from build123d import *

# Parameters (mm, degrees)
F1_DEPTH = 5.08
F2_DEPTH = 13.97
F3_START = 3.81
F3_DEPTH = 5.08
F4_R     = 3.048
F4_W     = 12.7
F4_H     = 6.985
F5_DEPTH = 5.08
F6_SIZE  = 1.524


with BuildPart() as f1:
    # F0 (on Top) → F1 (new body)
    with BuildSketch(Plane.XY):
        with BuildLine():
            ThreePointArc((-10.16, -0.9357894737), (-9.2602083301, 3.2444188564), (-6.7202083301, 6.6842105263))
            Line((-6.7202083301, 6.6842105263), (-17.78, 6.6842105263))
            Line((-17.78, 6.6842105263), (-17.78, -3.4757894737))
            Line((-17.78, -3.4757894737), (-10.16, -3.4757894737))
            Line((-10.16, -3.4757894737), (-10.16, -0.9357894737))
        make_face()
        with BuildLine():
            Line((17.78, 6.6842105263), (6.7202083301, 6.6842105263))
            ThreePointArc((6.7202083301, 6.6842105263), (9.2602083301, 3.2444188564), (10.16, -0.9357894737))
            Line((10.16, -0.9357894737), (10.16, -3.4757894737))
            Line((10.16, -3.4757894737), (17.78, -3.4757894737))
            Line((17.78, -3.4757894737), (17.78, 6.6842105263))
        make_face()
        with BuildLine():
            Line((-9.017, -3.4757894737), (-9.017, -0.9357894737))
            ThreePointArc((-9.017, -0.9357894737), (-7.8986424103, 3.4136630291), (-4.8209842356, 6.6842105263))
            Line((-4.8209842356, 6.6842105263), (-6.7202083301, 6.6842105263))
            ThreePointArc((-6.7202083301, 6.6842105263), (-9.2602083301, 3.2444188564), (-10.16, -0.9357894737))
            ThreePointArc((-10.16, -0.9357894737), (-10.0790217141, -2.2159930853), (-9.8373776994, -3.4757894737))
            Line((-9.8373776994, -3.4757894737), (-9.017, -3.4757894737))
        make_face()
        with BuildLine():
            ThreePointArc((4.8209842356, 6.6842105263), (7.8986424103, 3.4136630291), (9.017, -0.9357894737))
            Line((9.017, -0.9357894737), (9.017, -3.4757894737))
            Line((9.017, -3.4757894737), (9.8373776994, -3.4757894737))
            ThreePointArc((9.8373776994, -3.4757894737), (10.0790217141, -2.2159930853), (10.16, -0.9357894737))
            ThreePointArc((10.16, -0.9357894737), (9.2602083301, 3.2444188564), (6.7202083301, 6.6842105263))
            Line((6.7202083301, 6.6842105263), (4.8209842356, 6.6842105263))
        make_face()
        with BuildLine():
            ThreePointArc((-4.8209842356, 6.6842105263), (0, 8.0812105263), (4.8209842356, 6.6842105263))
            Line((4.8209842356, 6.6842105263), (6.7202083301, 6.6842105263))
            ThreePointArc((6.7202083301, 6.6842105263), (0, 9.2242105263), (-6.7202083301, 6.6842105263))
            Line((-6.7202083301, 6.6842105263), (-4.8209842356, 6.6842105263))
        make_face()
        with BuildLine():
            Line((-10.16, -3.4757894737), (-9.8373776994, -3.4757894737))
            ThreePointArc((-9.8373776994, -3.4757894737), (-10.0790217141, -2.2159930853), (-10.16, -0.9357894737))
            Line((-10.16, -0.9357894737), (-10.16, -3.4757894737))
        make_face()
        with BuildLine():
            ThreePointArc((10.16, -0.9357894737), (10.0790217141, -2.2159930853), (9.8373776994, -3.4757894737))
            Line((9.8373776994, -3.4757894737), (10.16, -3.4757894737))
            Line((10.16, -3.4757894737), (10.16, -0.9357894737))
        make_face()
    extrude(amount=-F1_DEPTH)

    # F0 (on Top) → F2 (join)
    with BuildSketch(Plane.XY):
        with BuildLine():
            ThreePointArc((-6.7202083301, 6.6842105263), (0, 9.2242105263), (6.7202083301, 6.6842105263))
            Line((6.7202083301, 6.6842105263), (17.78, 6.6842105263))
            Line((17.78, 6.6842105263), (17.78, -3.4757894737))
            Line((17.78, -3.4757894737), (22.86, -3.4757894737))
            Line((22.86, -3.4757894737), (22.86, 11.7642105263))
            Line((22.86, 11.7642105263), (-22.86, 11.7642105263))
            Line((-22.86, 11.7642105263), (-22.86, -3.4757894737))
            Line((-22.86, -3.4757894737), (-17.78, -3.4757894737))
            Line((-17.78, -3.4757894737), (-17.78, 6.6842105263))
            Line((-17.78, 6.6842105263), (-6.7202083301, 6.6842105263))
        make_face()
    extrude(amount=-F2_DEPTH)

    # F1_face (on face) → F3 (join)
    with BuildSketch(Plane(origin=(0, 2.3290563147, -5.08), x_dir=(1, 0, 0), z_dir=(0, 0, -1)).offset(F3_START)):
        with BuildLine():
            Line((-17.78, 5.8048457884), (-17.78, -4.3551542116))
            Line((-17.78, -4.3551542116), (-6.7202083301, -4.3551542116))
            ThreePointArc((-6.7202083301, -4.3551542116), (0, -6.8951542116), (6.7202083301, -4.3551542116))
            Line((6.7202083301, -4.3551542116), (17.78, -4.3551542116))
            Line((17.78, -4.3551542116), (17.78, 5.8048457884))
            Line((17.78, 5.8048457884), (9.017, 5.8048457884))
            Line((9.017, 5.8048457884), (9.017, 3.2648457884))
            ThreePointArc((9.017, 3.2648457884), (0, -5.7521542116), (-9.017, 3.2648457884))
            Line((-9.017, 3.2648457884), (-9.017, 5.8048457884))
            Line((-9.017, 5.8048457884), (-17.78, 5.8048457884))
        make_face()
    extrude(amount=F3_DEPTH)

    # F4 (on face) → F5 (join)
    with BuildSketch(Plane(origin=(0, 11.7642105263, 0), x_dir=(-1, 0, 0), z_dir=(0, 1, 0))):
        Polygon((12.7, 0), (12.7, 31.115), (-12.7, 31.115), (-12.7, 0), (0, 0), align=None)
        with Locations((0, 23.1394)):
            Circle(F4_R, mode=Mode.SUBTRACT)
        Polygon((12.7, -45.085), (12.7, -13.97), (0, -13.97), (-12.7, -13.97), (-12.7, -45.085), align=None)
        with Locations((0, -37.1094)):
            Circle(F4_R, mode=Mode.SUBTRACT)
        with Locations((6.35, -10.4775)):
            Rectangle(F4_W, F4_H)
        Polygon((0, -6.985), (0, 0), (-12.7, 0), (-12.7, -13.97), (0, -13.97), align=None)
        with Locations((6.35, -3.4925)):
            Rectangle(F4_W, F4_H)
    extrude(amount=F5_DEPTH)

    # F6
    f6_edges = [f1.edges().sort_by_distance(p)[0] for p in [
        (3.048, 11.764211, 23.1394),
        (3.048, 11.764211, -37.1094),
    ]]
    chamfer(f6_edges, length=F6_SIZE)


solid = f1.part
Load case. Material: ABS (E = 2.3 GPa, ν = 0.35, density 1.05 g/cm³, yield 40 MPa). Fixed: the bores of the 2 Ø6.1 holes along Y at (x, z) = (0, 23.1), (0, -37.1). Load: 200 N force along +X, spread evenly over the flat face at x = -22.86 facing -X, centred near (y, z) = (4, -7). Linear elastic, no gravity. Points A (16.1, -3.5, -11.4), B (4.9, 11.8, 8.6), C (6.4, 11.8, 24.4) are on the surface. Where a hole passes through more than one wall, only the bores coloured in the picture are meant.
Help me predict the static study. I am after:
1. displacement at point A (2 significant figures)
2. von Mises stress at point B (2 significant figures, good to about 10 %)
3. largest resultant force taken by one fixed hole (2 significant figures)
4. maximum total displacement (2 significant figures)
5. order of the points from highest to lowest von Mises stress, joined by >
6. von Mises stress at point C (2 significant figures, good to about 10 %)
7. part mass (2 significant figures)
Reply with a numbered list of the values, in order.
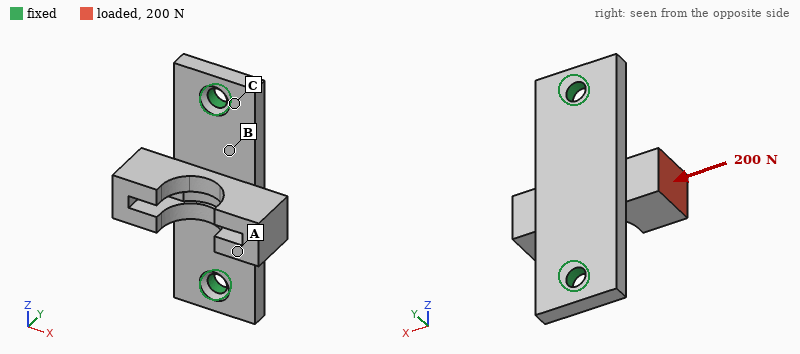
1. 0.66 mm
2. 8.4 MPa
3. 100 N
4. 0.96 mm
5. B > C > A
6. 5.3 MPa
7. 17 g
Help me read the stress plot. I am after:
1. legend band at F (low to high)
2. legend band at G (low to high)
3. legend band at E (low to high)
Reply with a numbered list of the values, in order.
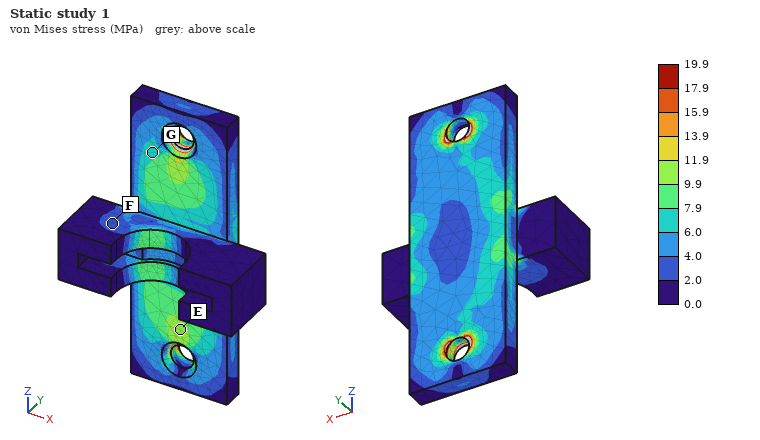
1. 2.0 to 4.0 MPa
2. 6.0 to 7.9 MPa
3. 9.9 to 11.9 MPa
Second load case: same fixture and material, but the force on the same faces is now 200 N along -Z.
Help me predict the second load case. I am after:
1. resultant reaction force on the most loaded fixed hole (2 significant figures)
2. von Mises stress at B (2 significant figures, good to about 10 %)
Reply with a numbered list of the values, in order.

1. 140 N
2. 2.1 MPa
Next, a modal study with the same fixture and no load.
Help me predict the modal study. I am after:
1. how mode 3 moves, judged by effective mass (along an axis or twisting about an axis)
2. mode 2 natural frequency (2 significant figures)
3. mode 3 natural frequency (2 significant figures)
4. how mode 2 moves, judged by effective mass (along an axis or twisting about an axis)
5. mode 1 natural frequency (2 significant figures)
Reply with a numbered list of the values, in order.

1. along Z
2. 1300 Hz
3. 2500 Hz
4. along Y
5. 860 Hz
